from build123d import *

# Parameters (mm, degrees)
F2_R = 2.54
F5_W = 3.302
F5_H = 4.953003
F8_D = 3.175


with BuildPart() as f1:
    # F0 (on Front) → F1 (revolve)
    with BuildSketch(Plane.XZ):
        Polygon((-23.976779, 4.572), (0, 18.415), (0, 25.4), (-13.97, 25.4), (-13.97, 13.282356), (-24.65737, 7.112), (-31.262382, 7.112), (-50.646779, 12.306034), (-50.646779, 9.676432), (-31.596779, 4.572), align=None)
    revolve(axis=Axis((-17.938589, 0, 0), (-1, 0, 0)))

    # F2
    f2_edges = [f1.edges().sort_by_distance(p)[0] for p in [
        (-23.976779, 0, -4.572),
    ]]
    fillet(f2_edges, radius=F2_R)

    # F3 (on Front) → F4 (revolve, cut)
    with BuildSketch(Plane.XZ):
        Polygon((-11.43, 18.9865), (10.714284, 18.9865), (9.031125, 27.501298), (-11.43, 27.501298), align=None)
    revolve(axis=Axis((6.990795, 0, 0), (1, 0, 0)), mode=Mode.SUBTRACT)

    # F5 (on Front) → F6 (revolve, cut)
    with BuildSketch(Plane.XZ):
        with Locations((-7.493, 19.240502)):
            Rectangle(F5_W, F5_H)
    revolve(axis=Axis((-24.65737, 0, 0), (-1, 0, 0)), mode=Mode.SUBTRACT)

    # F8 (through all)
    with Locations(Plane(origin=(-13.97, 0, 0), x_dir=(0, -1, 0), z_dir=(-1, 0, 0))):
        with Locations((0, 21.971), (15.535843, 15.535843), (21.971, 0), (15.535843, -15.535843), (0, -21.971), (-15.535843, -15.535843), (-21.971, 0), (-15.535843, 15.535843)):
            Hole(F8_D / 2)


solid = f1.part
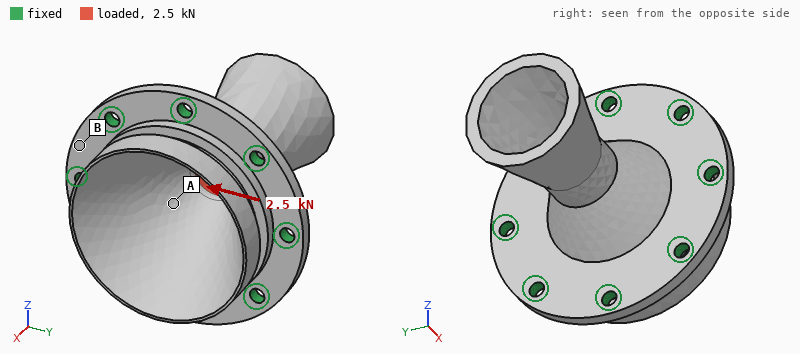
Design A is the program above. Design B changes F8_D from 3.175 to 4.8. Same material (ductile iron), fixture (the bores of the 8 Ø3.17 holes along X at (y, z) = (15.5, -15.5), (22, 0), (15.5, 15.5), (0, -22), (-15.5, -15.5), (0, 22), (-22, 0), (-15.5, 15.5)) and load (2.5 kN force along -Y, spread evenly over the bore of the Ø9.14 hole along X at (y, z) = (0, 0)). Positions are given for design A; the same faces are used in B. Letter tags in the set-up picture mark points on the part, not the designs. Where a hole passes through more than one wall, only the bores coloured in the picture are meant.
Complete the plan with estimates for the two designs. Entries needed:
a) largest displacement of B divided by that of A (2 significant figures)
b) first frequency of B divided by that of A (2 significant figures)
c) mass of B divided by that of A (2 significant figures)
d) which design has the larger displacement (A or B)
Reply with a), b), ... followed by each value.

a) 0.90
b) 1.0
c) 0.98
d) A
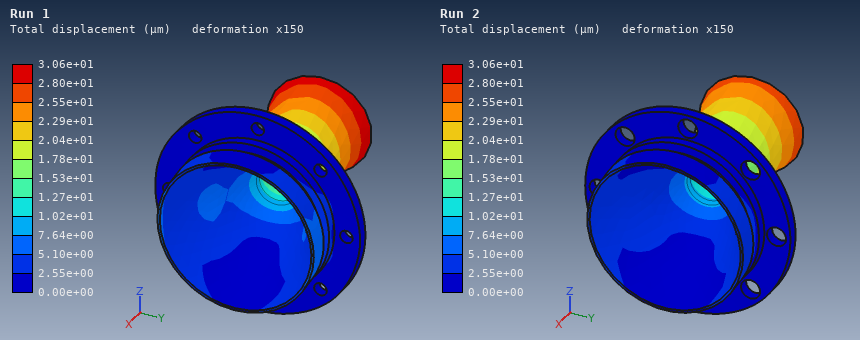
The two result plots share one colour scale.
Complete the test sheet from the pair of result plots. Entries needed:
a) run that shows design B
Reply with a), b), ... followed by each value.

a) Run 2
